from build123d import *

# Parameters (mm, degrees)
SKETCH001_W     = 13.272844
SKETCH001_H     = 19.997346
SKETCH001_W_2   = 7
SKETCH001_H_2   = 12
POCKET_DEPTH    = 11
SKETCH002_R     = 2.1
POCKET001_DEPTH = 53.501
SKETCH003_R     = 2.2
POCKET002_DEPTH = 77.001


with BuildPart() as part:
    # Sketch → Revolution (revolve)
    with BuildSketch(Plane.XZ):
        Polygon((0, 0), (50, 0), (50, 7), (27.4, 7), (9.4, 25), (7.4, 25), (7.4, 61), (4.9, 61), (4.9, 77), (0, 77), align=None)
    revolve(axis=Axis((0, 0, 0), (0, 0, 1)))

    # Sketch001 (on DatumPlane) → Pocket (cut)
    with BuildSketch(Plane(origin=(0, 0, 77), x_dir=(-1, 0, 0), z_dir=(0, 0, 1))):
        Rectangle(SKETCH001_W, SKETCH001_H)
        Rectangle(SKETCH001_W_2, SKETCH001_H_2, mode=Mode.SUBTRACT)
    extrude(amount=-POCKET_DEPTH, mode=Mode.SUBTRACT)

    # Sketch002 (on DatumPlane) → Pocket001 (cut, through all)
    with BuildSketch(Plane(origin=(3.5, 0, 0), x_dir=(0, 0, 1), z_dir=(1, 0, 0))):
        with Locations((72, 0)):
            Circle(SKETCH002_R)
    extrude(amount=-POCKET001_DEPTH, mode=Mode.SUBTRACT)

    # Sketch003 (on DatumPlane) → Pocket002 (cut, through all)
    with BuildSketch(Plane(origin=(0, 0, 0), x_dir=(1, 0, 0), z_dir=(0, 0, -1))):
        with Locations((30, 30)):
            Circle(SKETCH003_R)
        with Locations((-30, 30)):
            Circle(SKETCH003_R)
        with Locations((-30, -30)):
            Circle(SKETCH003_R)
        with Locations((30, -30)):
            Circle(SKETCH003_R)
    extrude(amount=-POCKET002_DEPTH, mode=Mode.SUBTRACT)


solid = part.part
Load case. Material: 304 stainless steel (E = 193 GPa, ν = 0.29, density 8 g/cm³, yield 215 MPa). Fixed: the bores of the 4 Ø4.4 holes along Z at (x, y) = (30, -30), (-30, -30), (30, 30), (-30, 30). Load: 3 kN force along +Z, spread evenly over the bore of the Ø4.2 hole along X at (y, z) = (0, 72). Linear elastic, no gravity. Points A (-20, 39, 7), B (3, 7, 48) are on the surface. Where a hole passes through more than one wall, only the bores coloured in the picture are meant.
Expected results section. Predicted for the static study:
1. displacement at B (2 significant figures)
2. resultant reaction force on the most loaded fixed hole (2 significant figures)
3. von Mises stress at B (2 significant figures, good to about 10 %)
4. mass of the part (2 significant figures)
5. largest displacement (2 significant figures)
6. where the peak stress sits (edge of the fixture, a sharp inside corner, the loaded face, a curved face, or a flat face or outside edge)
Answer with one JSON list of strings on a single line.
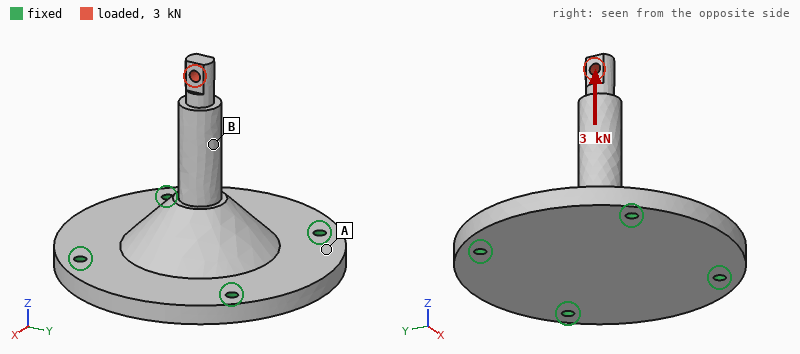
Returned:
["8.0 µm", "820 N", "17 MPa", "660 g", "14 µm", "the loaded face"]
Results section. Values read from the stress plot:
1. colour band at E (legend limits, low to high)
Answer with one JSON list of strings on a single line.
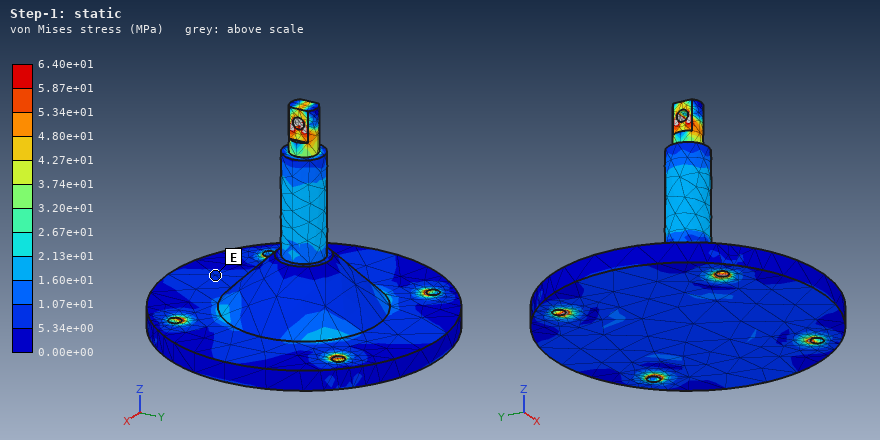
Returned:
["5.34e+00 to 1.07e+01 MPa"]
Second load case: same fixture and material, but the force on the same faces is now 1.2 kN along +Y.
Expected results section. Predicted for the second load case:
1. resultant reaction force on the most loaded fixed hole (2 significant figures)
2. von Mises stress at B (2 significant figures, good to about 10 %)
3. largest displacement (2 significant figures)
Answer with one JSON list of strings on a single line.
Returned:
["830 N", "87 MPa", "0.17 mm"]
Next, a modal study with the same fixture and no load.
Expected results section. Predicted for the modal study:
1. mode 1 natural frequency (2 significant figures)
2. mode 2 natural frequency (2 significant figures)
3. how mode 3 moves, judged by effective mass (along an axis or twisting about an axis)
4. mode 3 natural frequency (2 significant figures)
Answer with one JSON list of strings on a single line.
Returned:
["4000 Hz", "4000 Hz", "along Z", "5700 Hz"]
